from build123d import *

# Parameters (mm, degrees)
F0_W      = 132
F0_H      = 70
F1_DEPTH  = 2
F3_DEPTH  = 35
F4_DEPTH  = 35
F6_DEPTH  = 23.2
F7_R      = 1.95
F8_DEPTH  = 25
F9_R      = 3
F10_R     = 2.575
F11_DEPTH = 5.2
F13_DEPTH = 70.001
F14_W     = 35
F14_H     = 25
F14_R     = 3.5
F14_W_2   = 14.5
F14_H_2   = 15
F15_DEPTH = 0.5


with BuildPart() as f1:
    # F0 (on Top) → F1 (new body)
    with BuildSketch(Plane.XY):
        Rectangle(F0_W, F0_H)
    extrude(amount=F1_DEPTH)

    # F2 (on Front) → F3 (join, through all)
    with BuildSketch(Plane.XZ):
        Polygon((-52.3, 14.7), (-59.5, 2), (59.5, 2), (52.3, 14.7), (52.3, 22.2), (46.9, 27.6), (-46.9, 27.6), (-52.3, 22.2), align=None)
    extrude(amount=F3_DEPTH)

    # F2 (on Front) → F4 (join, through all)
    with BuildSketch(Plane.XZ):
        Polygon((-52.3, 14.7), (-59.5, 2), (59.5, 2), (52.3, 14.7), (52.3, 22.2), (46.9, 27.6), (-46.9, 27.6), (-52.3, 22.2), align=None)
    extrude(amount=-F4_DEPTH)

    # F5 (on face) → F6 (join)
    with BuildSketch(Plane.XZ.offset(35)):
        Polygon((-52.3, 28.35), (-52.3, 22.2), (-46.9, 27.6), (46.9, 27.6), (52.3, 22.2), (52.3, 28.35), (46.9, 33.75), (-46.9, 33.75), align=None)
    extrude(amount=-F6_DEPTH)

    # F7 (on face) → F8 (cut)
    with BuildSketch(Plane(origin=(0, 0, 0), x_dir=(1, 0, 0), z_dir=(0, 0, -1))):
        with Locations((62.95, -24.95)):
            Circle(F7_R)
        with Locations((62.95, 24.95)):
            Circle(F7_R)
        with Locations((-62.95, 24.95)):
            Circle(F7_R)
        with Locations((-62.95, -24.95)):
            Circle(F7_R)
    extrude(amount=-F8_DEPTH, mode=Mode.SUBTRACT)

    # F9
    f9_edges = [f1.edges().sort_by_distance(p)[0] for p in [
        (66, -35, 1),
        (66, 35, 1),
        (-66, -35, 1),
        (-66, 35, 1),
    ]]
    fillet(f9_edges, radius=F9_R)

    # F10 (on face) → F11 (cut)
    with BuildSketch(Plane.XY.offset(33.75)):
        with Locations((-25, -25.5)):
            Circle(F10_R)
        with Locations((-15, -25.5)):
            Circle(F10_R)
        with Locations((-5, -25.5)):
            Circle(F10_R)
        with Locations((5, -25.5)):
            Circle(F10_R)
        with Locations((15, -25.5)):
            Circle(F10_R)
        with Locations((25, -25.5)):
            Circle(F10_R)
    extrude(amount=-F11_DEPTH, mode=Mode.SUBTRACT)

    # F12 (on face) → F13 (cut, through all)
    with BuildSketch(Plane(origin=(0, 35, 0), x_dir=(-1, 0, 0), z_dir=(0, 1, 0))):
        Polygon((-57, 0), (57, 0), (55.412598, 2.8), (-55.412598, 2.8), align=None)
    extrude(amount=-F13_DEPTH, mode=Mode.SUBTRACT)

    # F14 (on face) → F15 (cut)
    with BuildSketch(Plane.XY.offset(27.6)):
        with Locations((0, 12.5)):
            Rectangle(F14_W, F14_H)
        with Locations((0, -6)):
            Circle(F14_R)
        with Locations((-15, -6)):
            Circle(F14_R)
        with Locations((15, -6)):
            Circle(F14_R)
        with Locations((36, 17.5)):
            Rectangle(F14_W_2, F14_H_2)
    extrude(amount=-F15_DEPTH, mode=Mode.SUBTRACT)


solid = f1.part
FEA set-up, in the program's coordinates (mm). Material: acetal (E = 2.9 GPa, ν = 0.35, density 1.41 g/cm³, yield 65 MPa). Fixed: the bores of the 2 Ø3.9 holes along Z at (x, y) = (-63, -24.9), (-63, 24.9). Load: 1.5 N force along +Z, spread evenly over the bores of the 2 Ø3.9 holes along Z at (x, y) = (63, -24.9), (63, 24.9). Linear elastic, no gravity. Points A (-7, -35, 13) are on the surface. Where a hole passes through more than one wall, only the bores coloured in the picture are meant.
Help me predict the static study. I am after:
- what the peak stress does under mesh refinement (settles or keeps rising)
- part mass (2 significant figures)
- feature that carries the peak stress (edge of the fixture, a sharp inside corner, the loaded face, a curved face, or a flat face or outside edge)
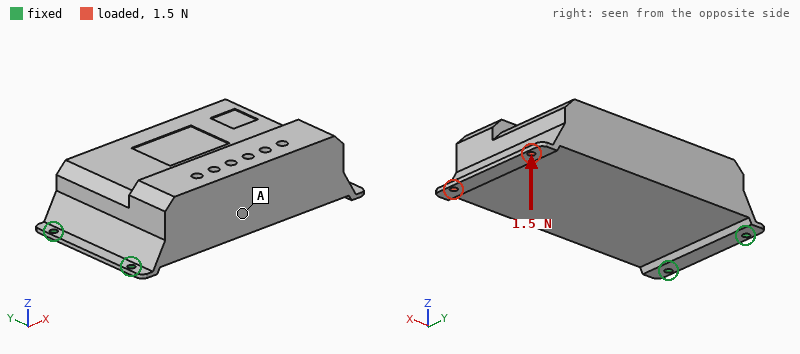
keeps rising
280 g
edge of the fixture
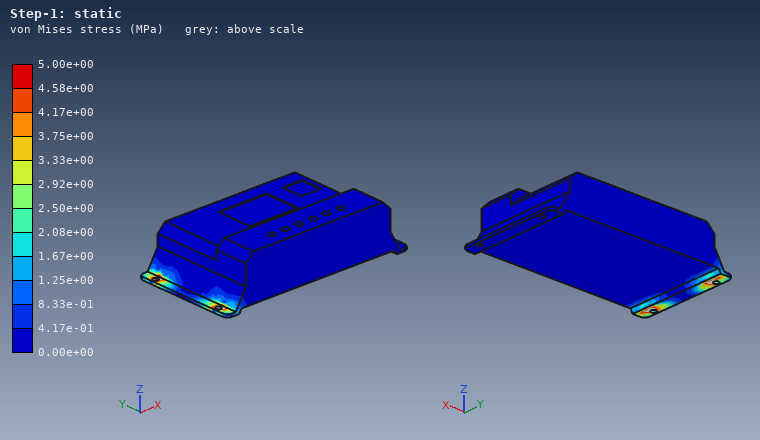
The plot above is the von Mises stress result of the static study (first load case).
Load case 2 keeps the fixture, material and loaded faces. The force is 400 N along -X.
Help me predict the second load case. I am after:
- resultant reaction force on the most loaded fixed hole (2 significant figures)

200 N
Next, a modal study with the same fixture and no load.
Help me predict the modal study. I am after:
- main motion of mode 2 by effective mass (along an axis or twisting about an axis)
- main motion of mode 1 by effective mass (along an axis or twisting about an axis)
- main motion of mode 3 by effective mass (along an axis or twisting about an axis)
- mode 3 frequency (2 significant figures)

along Y
along Z
along Y
520 Hz
